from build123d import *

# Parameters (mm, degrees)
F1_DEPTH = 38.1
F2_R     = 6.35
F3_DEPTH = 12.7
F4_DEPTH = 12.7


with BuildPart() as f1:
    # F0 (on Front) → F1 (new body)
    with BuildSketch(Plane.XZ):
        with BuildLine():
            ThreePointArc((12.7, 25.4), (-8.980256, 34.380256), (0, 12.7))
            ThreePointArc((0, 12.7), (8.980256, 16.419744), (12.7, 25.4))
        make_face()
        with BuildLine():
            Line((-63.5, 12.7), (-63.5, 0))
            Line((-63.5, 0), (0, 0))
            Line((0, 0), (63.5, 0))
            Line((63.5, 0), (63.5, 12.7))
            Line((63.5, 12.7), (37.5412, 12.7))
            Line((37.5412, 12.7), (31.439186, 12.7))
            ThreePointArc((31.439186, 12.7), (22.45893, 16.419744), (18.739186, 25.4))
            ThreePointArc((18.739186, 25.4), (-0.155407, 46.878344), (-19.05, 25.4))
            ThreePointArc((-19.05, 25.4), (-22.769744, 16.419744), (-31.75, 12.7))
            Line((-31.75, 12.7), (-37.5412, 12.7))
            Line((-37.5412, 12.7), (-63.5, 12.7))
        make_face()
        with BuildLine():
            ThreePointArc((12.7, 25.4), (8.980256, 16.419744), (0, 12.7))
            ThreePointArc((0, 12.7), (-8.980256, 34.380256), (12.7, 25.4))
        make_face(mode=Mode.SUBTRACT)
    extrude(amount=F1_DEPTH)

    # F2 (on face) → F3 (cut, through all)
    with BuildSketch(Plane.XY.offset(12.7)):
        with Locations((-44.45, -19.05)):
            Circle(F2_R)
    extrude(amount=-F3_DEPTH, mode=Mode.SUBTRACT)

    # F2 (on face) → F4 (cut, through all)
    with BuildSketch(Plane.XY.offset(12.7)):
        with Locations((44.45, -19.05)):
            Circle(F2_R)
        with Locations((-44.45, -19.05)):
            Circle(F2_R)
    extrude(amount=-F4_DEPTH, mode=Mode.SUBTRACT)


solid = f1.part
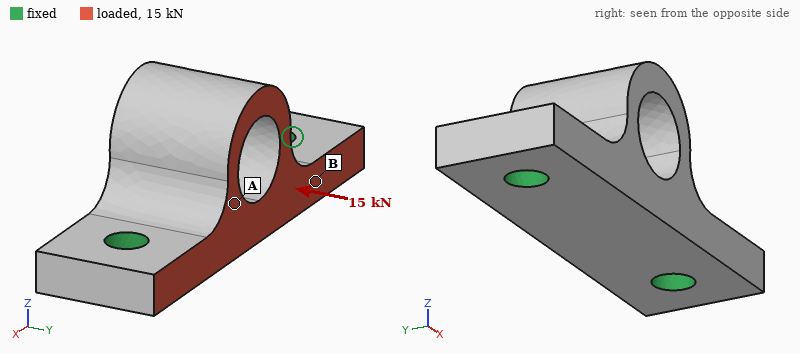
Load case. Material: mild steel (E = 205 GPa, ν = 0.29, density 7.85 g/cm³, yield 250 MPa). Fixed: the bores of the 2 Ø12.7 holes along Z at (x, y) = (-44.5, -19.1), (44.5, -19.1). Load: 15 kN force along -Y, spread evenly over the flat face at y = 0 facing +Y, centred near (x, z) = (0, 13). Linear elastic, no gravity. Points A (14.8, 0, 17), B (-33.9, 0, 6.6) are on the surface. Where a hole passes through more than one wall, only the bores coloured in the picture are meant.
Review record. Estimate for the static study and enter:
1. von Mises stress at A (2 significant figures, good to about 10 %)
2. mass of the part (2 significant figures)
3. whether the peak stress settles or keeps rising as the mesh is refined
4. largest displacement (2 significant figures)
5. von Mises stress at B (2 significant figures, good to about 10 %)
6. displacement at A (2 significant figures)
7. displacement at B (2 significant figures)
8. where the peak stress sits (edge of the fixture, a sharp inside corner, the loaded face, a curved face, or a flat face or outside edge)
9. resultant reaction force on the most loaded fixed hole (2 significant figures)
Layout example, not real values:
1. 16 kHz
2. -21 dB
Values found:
1. 15 MPa
2. 670 g
3. keeps rising
4. 32 µm
5. 37 MPa
6. 15 µm
7. 6.0 µm
8. edge of the fixture
9. 7.5 kN
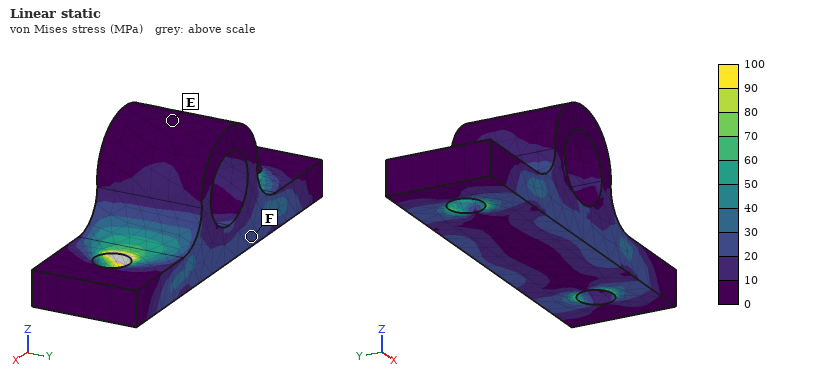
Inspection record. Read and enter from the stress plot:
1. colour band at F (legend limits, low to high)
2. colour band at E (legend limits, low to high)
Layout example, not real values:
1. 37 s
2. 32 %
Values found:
1. 20 to 30 MPa
2. 0 to 10 MPa
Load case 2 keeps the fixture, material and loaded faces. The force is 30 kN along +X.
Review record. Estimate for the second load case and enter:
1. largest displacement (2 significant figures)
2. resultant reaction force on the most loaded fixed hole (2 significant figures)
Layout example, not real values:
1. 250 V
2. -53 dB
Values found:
1. 30 µm
2. 16 kN
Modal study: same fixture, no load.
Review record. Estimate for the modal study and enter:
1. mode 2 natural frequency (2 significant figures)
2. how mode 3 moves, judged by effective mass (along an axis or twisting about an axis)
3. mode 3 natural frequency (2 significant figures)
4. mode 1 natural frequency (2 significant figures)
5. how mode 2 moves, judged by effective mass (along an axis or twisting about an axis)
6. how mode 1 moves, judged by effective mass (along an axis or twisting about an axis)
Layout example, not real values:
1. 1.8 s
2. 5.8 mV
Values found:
1. 7300 Hz
2. along X
3. 9400 Hz
4. 4800 Hz
5. along Z
6. along Y
